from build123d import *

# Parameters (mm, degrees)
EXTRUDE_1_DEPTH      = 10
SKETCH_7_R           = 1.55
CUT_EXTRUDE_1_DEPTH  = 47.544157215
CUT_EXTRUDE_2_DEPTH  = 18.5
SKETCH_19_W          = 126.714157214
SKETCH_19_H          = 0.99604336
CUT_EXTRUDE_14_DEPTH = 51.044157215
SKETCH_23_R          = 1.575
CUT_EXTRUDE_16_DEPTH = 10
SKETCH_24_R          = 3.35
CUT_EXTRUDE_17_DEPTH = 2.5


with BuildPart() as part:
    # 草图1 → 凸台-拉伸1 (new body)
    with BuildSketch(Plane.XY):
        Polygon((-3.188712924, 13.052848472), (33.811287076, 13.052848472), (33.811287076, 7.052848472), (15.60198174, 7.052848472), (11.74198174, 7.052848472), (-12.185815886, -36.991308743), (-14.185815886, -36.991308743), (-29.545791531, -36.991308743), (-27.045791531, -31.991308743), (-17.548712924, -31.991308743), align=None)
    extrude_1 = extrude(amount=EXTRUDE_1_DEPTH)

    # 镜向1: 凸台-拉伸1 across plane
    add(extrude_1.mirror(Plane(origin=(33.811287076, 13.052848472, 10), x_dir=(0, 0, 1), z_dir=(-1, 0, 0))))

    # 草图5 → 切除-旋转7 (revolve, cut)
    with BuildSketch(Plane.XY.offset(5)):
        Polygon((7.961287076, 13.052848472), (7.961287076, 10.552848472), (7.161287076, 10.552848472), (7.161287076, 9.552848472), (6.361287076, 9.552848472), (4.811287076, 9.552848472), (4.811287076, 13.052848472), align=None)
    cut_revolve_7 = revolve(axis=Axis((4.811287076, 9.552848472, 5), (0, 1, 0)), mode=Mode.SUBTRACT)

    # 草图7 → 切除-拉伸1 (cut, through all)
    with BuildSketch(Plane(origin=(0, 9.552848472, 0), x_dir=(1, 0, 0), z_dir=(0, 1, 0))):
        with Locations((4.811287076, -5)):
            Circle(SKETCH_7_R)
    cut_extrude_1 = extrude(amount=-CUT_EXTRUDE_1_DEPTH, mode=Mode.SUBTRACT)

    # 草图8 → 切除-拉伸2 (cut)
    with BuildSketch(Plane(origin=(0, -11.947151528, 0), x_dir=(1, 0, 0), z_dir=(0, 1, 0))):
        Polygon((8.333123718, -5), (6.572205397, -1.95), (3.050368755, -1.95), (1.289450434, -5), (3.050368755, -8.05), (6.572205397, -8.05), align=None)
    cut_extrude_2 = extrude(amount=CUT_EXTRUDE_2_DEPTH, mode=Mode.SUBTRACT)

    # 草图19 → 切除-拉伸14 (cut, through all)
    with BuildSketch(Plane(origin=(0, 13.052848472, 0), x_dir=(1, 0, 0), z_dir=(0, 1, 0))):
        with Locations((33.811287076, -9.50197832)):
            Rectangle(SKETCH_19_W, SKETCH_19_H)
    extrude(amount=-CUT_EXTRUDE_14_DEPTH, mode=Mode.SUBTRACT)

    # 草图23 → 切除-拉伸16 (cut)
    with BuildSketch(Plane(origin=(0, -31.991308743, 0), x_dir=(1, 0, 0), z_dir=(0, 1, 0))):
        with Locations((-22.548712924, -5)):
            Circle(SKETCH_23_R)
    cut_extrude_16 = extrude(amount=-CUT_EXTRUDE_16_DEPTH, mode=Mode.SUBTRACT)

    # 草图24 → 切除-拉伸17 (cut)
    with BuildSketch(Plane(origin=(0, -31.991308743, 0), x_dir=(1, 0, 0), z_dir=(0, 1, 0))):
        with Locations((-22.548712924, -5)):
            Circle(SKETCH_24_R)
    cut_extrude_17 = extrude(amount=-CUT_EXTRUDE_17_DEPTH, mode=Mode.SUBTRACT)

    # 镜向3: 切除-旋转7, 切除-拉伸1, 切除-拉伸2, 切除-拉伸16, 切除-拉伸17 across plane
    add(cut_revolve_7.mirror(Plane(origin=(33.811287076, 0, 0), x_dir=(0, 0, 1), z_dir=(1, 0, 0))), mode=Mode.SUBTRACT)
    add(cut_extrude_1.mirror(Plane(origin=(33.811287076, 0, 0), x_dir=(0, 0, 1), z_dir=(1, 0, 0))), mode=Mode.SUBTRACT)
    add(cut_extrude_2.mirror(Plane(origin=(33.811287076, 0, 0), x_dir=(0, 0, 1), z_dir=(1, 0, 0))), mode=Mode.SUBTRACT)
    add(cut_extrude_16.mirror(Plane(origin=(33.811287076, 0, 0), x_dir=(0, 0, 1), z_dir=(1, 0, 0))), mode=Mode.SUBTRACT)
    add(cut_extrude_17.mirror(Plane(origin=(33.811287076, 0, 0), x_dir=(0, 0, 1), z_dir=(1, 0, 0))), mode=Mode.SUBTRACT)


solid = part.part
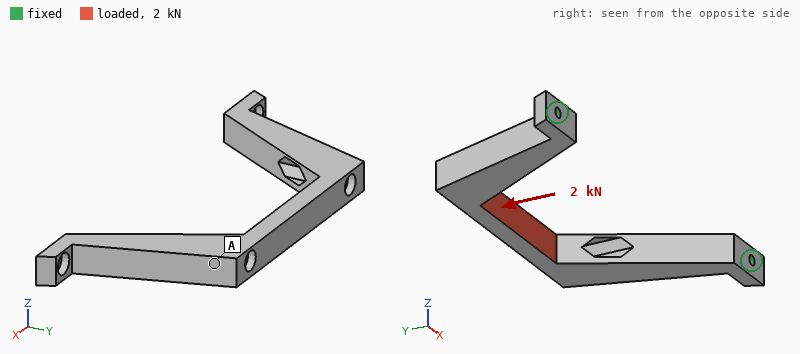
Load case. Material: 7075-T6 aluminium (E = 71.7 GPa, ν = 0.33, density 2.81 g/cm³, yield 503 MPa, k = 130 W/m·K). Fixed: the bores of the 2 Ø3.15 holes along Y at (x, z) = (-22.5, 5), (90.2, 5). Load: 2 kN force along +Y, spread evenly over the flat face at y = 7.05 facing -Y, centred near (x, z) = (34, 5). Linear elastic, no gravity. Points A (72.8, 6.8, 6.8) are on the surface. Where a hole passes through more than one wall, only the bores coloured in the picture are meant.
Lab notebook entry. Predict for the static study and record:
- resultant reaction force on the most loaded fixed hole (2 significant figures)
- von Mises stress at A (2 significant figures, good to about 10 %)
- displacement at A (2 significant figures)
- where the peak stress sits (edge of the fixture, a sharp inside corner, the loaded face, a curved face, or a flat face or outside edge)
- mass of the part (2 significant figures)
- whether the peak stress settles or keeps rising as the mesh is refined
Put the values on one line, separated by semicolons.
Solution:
1.3 kN; 23 MPa; 0.026 mm; edge of the fixture; 37 g; keeps rising
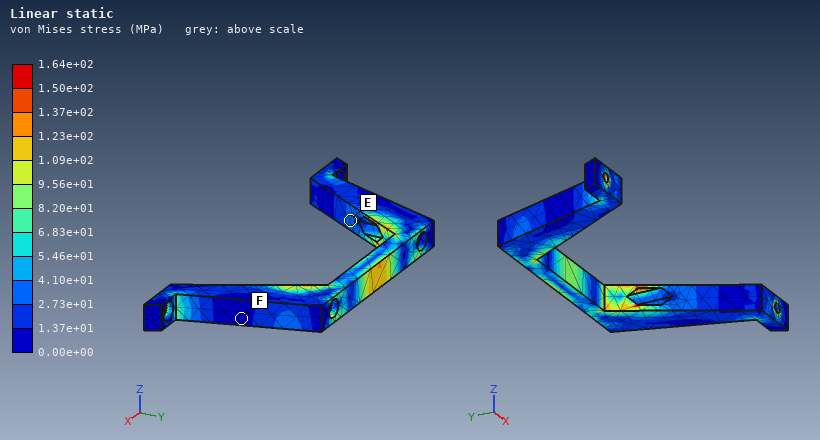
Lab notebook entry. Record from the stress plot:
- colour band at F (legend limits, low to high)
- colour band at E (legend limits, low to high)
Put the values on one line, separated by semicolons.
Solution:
0.00e+00 to 1.37e+01 MPa; 2.73e+01 to 4.10e+01 MPa
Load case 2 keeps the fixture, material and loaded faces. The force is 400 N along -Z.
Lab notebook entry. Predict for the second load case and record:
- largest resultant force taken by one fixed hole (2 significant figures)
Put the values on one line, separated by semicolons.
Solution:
200 N
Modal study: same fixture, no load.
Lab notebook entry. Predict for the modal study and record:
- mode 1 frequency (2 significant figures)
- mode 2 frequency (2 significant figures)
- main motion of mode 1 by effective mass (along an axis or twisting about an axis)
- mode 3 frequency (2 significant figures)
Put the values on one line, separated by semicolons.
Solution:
790 Hz; 2100 Hz; along Z; 2100 Hz
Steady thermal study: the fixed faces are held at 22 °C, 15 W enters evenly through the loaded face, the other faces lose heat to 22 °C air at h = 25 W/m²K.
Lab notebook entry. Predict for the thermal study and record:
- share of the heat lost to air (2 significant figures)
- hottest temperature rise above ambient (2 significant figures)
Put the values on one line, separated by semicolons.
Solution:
28 %; 50 K
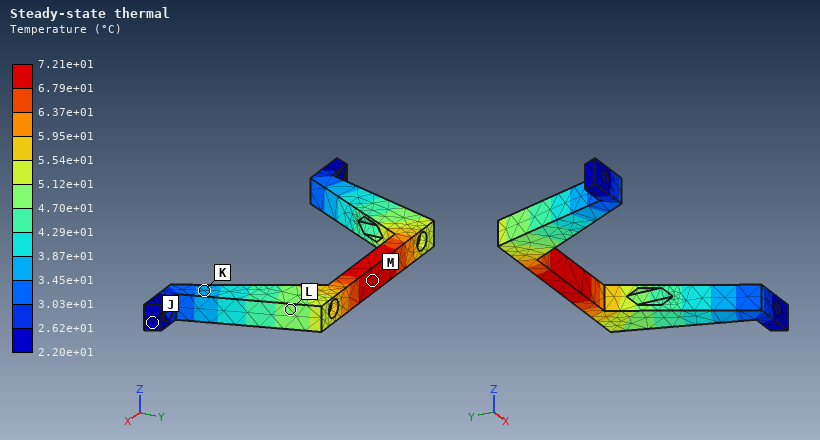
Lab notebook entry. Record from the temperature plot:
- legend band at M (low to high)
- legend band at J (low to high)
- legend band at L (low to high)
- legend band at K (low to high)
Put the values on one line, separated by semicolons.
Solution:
6.79e+01 to 7.21e+01 °C; 2.20e+01 to 2.62e+01 °C; 4.70e+01 to 5.12e+01 °C; 3.45e+01 to 3.87e+01 °C
